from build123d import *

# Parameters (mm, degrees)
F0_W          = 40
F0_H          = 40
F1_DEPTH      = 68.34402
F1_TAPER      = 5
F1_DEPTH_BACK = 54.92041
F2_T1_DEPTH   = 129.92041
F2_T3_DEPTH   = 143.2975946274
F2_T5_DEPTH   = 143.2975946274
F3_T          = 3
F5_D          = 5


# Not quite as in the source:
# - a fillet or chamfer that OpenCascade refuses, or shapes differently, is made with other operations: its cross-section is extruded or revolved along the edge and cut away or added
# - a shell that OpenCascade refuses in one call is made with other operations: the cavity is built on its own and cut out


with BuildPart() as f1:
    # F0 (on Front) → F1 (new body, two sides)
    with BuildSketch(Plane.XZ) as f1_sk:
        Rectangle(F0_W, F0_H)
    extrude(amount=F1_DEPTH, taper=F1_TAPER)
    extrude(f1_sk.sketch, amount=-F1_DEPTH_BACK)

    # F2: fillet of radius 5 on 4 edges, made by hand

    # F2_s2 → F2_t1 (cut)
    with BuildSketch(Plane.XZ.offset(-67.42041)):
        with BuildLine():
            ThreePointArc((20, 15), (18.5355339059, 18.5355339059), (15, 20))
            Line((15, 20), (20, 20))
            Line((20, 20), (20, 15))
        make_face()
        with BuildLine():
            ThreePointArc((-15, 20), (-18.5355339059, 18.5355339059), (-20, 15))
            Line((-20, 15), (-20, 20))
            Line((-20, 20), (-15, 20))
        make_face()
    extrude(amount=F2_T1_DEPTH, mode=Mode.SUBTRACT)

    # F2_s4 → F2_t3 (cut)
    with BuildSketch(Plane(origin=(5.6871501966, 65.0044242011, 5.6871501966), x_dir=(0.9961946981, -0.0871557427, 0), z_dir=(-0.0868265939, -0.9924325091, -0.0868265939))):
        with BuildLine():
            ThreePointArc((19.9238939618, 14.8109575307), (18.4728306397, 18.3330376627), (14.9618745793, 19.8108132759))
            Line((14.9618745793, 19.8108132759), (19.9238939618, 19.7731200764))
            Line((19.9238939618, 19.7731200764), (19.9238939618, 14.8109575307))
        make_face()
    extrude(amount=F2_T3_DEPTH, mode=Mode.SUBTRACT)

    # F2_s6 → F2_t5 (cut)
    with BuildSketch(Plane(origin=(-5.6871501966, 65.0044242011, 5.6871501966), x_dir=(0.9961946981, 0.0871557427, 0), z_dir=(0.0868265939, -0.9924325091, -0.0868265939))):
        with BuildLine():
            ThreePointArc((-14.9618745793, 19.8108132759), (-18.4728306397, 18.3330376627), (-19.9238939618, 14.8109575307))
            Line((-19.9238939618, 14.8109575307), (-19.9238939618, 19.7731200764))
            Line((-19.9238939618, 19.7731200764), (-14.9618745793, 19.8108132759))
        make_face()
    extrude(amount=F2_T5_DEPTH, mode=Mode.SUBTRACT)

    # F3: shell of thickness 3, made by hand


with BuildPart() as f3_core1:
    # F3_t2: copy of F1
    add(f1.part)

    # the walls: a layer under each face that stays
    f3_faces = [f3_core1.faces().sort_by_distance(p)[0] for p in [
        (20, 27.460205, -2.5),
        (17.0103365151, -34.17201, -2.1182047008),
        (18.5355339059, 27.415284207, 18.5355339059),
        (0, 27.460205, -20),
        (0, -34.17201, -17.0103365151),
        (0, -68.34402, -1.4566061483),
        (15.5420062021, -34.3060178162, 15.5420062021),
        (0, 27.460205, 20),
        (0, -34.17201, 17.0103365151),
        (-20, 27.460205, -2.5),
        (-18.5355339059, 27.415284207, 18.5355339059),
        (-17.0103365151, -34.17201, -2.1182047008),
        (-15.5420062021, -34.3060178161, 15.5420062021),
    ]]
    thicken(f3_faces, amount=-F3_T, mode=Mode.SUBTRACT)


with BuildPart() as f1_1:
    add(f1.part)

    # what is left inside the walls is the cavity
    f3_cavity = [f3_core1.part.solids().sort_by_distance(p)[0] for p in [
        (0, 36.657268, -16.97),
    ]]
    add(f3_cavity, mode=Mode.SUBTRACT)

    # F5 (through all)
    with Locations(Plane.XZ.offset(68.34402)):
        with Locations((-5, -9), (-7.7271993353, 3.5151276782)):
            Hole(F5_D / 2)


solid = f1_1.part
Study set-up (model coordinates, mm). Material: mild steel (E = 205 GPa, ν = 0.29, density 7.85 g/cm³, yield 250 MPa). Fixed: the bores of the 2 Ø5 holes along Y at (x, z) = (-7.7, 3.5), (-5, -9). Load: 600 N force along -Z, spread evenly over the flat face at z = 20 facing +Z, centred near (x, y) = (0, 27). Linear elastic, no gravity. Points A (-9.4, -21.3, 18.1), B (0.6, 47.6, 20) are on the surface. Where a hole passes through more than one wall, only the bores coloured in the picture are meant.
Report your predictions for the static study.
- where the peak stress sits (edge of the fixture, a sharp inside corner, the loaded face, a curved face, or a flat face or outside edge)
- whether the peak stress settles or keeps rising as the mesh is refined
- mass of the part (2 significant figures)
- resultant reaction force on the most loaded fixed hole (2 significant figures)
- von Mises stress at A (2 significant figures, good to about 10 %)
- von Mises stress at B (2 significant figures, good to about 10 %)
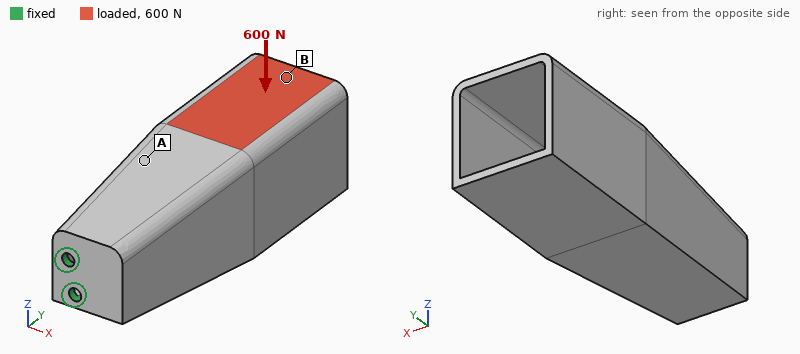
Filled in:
edge of the fixture
keeps rising
390 g
3.0 kN
11 MPa
21 MPa
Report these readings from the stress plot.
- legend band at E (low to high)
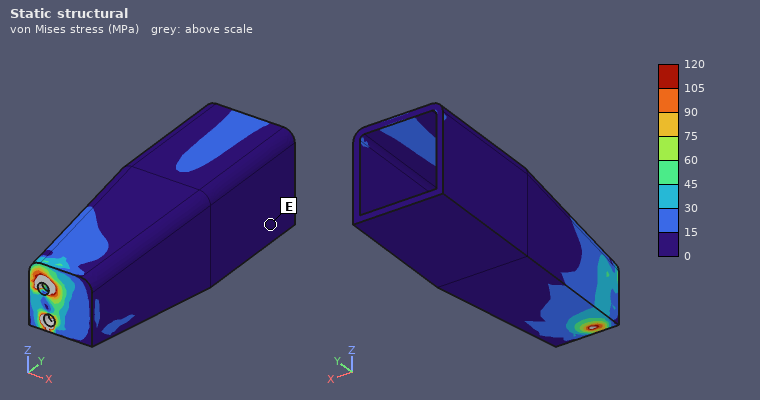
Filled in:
0 to 15 MPa
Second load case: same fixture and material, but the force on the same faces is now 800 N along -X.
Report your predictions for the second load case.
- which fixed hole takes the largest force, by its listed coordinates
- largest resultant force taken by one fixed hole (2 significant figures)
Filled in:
(-7.7, 3.5)
1.9 kN
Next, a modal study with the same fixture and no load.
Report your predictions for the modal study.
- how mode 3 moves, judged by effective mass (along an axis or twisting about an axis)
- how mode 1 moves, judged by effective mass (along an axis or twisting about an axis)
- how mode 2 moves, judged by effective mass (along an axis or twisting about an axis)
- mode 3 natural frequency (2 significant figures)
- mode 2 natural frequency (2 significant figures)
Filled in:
twisting about Y
along X
along Z
3300 Hz
790 Hz
